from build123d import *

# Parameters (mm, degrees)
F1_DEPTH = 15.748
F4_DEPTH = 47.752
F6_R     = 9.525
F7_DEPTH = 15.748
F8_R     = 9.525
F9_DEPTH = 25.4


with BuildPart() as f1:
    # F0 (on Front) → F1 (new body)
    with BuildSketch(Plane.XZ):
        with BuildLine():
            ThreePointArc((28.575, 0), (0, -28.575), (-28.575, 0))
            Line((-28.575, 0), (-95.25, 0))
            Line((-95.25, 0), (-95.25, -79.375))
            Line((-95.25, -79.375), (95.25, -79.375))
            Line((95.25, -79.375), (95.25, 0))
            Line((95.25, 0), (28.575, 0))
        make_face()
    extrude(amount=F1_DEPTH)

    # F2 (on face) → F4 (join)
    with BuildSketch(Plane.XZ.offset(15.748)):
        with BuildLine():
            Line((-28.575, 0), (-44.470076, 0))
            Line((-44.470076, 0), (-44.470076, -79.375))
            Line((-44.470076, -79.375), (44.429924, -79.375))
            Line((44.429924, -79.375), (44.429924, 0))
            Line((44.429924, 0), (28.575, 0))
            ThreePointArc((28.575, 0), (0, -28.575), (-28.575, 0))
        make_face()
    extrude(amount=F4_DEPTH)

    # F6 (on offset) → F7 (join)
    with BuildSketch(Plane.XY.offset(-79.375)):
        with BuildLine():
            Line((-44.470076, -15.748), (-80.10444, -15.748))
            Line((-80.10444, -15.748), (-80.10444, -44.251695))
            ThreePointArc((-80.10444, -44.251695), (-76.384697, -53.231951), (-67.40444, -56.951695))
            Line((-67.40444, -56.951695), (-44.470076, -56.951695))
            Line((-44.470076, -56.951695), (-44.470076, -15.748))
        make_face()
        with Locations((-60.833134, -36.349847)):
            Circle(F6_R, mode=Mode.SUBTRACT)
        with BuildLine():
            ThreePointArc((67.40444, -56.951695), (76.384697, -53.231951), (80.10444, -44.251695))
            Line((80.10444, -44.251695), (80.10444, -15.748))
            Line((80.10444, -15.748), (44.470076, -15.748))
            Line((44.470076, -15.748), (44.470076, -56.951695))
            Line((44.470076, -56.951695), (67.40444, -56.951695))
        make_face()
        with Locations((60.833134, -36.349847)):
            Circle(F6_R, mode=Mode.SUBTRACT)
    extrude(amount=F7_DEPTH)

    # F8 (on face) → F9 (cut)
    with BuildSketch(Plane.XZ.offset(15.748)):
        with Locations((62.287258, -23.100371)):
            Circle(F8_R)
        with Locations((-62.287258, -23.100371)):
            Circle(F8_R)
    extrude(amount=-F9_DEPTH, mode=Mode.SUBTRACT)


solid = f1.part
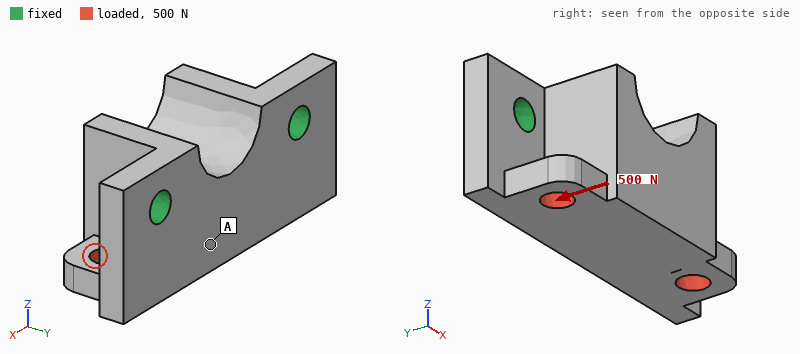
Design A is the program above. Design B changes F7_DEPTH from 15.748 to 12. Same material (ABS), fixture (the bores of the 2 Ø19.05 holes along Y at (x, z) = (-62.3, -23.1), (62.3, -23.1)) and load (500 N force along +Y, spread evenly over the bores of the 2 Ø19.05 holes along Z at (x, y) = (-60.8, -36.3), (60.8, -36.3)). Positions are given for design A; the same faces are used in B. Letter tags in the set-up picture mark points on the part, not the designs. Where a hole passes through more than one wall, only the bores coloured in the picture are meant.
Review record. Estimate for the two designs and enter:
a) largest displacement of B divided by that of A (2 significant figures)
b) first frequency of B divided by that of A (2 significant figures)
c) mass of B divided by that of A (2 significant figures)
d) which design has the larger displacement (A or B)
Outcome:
1.1
1.0
0.98
B
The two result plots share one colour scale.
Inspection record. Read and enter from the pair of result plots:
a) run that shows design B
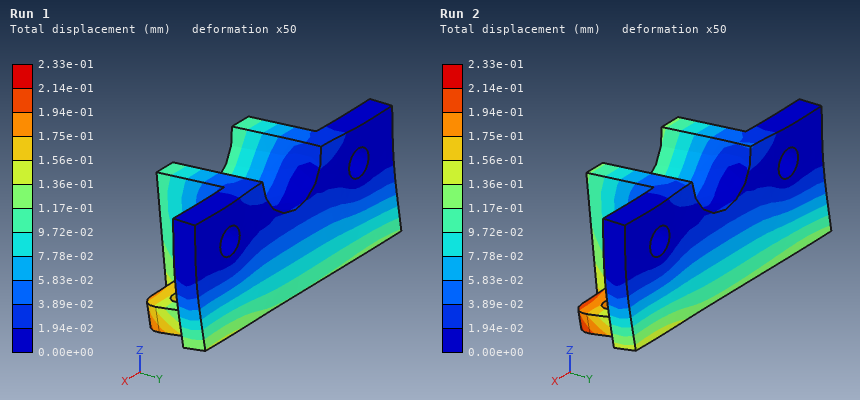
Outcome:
Run 2
